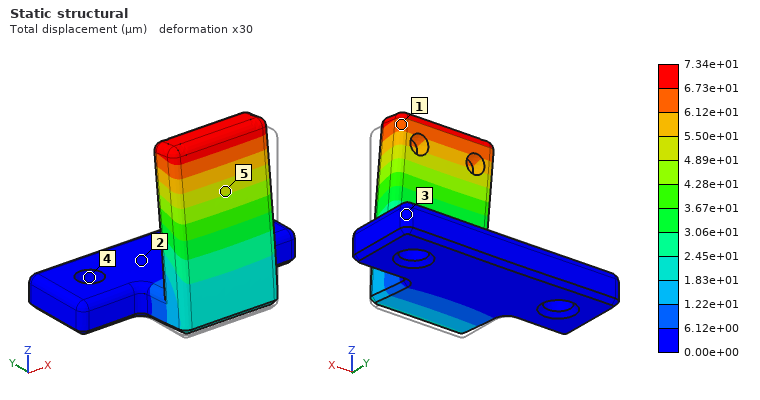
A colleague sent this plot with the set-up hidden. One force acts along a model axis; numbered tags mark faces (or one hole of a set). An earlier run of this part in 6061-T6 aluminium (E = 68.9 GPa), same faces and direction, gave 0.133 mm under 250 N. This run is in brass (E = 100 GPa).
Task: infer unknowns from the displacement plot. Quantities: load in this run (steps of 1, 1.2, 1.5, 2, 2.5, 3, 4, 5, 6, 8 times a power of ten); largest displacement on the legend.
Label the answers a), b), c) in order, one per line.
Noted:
a) 200 N
b) 7.34e+01 µm
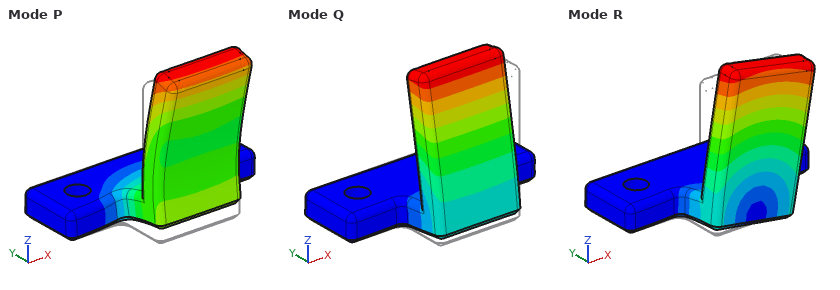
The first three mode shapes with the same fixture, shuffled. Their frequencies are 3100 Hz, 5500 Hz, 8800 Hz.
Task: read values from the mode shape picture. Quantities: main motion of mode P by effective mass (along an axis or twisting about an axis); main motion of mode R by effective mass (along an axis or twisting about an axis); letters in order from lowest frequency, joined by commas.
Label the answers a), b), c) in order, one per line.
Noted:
a) along Z
b) along X
c) Q, R, P
